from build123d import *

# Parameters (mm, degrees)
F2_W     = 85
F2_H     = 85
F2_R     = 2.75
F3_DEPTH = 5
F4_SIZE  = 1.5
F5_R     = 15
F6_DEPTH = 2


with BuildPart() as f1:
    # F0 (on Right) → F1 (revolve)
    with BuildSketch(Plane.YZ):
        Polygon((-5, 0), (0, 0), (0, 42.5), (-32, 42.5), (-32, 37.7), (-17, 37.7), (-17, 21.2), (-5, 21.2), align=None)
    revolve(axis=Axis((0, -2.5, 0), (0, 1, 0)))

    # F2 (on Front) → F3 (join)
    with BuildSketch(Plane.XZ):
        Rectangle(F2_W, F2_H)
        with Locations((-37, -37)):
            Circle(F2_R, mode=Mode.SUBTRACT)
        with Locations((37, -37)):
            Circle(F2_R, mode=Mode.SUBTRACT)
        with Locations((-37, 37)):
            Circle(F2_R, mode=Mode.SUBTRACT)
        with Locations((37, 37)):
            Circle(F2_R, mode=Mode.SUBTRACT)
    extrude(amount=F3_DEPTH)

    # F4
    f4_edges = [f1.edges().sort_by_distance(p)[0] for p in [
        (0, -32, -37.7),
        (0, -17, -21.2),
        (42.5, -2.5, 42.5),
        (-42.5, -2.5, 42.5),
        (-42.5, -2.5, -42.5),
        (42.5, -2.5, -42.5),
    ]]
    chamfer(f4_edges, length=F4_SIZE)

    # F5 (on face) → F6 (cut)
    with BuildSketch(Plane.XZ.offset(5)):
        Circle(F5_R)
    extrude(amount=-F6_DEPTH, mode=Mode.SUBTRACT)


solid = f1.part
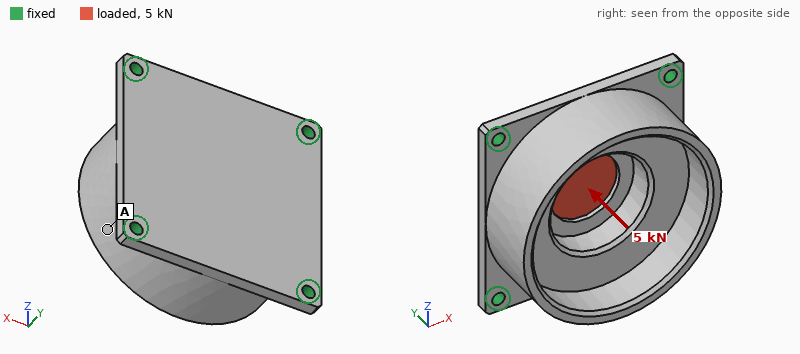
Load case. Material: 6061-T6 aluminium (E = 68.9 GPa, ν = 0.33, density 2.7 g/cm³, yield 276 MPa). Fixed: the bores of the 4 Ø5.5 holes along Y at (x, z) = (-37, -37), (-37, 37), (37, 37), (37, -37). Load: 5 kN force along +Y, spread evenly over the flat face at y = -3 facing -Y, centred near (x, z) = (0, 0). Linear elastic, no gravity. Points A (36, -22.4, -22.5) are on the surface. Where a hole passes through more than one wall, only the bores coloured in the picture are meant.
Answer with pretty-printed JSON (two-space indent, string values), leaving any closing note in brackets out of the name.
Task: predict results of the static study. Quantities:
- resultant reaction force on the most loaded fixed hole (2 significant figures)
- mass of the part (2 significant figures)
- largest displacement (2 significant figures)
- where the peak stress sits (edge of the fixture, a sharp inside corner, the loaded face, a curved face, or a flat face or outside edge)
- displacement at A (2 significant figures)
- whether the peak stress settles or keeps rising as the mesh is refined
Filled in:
{
  "resultant reaction force on the most loaded fixed hole": "1.5 kN",
  "mass of the part": "280 g",
  "largest displacement": "0.11 mm",
  "where the peak stress sits": "edge of the fixture",
  "displacement at A": "0.021 mm",
  "whether the peak stress settles or keeps rising as the mesh is refined": "keeps rising"
}
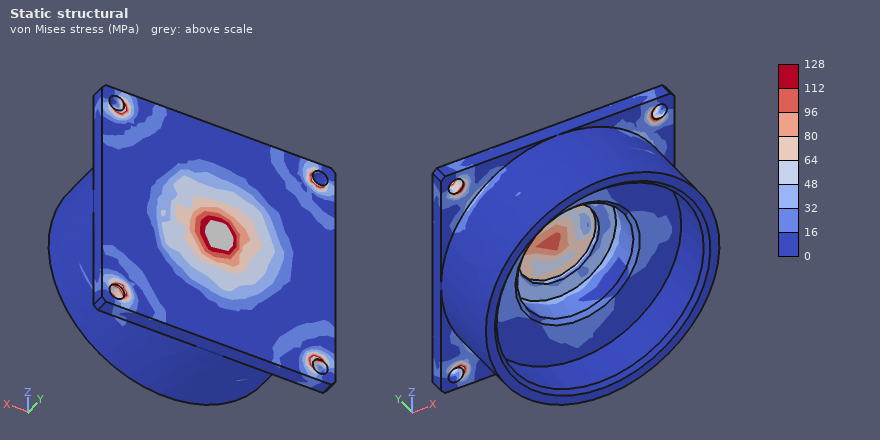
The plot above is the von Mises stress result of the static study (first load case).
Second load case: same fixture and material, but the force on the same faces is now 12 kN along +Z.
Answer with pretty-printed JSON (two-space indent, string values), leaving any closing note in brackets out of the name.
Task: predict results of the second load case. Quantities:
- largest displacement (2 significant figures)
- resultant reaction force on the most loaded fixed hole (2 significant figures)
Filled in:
{
  "largest displacement": "32 µm",
  "resultant reaction force on the most loaded fixed hole": "3.3 kN"
}
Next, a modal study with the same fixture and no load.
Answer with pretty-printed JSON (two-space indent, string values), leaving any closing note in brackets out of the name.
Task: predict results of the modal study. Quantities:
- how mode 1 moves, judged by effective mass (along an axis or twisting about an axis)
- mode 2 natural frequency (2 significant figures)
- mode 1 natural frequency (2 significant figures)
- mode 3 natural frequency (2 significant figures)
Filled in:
{
  "how mode 1 moves, judged by effective mass": "along Y",
  "mode 2 natural frequency": "5800 Hz",
  "mode 1 natural frequency": "4700 Hz",
  "mode 3 natural frequency": "5900 Hz"
}
